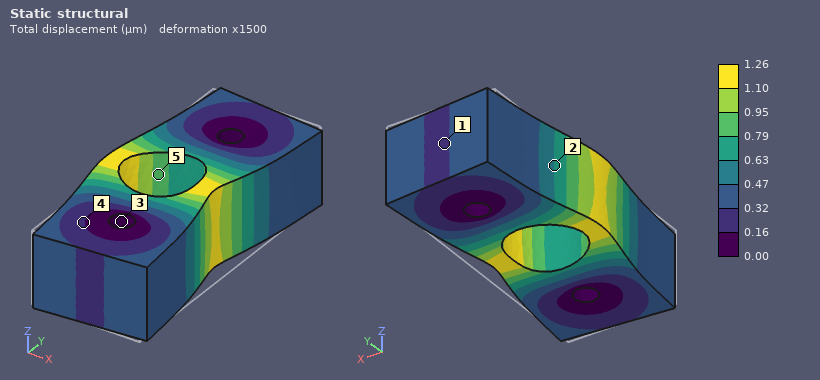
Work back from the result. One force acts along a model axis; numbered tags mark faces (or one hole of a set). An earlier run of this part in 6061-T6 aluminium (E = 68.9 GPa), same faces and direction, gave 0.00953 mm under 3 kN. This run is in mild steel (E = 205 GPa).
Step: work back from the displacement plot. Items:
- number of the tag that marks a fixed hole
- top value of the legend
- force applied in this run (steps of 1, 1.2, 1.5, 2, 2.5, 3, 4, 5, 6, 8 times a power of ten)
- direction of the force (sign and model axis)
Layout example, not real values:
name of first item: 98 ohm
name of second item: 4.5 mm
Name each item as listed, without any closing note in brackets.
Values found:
number of the tag that marks a fixed hole: 3
top value of the legend: 1.26 µm
force applied in this run: 1.2 kN
direction of the force: -X
